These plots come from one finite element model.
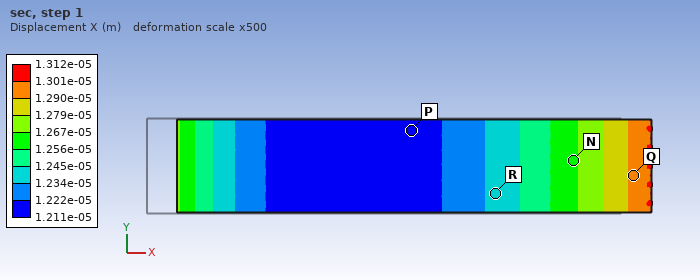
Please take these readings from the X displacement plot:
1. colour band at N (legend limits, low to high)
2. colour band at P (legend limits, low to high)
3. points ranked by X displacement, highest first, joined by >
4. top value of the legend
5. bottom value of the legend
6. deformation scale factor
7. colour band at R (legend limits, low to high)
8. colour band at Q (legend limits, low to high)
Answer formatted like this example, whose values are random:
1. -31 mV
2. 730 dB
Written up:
1. 1.256e-05 to 1.267e-05 m
2. 1.211e-05 to 1.222e-05 m
3. Q > N > R > P
4. 1.312e-05 m
5. 1.211e-05 m
6. 500
7. 1.234e-05 to 1.245e-05 m
8. 1.290e-05 to 1.301e-05 m
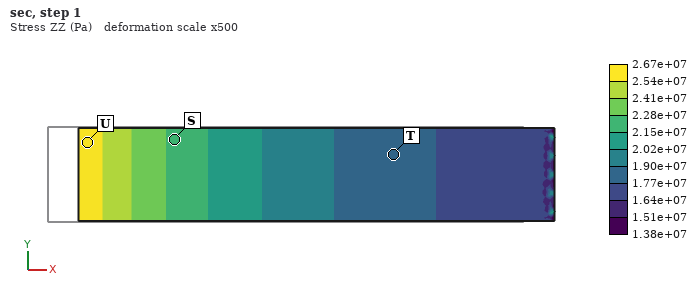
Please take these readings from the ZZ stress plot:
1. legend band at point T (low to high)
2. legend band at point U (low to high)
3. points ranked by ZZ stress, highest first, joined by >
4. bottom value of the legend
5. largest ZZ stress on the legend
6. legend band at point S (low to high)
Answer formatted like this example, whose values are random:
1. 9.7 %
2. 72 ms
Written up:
1. 1.77e+07 to 1.90e+07 Pa
2. 2.54e+07 to 2.67e+07 Pa
3. U > S > T
4. 1.38e+07 Pa
5. 2.67e+07 Pa
6. 2.15e+07 to 2.28e+07 Pa
